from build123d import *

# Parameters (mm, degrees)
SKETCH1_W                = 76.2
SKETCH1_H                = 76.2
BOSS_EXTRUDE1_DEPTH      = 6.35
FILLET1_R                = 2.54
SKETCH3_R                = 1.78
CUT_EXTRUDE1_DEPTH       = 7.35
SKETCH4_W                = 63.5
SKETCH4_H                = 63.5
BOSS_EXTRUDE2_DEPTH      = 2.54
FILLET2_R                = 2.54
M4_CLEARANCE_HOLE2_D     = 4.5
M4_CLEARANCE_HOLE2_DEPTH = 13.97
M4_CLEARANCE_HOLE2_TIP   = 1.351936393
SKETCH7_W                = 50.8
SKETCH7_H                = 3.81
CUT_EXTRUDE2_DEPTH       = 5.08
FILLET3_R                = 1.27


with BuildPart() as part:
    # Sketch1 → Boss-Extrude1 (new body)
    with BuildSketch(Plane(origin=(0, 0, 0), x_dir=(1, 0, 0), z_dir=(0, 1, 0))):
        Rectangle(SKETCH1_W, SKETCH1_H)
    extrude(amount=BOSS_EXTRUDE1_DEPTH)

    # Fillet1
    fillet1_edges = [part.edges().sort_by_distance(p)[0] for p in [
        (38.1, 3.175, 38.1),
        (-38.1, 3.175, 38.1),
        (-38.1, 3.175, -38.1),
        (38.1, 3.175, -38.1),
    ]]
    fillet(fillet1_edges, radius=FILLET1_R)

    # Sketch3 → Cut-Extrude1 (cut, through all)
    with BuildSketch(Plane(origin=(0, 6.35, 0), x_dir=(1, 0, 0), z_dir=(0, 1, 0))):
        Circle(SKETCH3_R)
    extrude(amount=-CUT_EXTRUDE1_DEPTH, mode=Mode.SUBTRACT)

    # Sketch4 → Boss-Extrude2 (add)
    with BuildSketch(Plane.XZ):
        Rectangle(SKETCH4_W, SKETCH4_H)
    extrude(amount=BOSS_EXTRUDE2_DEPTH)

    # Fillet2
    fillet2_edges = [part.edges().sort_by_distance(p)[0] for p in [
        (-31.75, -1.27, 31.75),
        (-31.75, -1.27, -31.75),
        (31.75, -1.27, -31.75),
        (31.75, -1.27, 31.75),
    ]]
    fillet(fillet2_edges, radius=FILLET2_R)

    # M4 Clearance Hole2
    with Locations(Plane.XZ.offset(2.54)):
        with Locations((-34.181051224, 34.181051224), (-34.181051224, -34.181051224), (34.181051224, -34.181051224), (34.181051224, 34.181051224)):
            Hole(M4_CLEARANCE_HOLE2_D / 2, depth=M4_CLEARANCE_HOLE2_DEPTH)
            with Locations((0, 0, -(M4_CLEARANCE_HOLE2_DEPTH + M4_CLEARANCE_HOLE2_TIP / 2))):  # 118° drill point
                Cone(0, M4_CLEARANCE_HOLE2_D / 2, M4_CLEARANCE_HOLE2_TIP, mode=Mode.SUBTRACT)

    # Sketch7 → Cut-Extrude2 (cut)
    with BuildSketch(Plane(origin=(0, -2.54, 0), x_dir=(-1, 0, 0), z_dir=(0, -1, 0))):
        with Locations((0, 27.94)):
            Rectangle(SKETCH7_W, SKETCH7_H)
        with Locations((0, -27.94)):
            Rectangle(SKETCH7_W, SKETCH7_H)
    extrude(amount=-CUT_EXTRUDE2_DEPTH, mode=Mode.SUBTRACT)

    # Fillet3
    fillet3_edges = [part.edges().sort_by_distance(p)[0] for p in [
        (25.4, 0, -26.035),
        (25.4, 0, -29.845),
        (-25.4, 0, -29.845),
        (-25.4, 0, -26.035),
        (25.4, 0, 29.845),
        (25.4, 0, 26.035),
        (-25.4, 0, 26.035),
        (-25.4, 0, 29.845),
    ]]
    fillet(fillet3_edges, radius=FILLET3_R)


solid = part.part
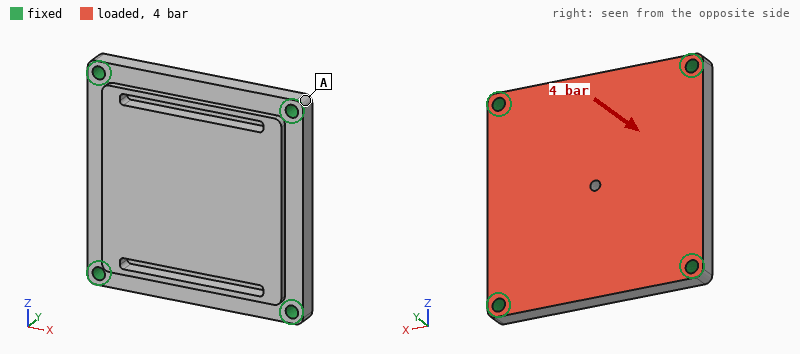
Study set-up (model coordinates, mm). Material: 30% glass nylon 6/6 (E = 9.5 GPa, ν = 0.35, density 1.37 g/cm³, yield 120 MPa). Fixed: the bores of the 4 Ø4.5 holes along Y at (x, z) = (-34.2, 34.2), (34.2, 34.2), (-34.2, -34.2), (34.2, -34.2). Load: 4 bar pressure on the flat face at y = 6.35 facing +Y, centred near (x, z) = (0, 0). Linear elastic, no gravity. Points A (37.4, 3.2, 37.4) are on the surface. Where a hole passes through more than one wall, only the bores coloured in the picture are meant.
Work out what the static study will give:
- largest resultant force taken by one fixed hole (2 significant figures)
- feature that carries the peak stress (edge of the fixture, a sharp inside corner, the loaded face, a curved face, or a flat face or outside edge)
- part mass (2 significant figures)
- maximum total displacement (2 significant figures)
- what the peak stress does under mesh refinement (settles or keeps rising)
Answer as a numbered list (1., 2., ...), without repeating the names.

1. 620 N
2. edge of the fixture
3. 61 g
4. 0.20 mm
5. keeps rising
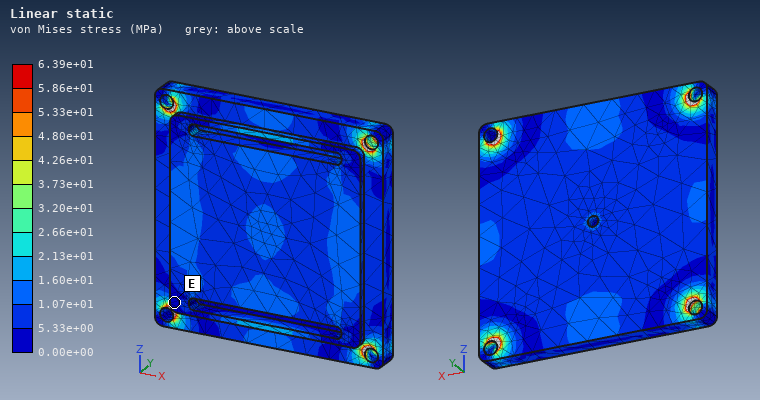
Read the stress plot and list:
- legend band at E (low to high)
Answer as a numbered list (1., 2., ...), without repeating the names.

1. 0.00e+00 to 5.33e+00 MPa
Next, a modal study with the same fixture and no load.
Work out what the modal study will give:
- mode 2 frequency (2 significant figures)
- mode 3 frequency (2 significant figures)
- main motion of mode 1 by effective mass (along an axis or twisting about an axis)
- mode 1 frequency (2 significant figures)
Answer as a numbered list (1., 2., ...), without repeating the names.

1. 4200 Hz
2. 4200 Hz
3. along Y
4. 2400 Hz
